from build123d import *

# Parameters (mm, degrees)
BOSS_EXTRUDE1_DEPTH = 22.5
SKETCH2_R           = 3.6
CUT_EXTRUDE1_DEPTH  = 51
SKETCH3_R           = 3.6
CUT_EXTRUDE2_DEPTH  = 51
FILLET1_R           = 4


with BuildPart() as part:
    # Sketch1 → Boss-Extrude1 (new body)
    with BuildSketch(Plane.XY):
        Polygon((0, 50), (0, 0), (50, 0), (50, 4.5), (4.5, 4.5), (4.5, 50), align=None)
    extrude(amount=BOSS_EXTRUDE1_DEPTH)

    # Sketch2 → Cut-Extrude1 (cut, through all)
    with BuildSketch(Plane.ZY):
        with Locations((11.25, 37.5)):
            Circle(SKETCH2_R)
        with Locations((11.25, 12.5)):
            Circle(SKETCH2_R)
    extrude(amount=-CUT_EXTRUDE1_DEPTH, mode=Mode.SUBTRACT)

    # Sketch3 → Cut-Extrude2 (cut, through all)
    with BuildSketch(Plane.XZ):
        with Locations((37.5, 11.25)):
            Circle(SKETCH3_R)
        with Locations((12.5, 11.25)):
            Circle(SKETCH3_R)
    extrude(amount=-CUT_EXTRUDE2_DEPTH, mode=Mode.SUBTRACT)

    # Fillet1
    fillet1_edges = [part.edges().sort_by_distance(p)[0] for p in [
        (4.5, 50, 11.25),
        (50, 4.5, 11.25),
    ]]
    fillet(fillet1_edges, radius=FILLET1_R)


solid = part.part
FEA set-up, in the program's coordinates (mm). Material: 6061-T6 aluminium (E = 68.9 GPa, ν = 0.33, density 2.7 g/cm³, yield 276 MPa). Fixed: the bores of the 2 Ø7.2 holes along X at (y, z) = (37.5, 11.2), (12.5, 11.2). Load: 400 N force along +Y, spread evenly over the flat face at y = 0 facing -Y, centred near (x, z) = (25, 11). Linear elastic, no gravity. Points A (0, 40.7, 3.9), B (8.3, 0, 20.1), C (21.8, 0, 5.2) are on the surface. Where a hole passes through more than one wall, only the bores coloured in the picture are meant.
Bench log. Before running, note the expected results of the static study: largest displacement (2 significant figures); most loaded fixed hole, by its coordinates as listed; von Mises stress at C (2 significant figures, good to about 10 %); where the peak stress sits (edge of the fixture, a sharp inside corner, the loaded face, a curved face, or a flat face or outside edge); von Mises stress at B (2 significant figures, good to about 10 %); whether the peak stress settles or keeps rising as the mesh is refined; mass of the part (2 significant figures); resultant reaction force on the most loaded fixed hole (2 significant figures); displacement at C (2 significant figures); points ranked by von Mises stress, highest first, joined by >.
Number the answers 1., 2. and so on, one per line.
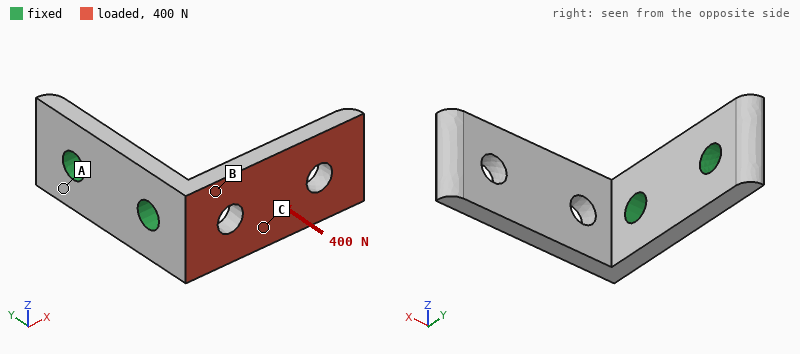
1. 0.76 mm
2. (12.5, 11.2)
3. 43 MPa
4. edge of the fixture
5. 110 MPa
6. keeps rising
7. 24 g
8. 380 N
9. 0.24 mm
10. B > C > A
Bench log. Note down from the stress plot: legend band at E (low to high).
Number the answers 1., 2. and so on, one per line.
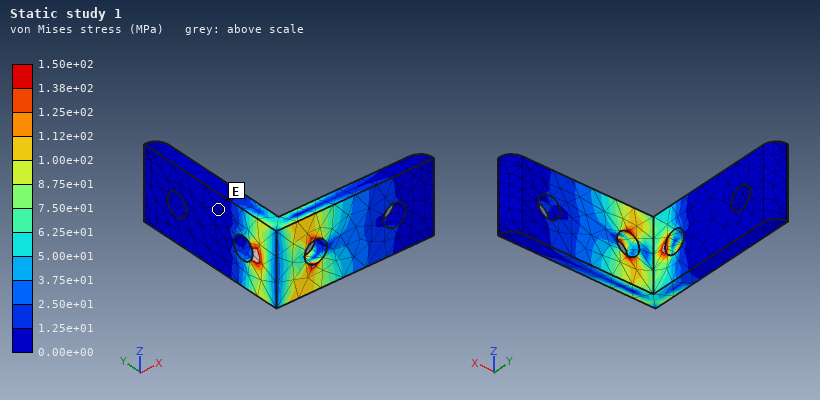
1. 0.00e+00 to 1.25e+01 MPa
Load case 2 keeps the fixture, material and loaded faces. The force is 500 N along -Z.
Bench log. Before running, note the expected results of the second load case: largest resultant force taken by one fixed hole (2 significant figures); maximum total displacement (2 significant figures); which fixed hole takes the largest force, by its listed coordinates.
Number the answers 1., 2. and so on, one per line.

1. 610 N
2. 0.20 mm
3. (12.5, 11.2)
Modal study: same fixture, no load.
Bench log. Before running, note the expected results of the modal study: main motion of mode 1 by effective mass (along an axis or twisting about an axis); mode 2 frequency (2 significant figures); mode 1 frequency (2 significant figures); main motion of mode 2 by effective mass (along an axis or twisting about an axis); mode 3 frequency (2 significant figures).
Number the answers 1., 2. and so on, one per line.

1. along Y
2. 2700 Hz
3. 1300 Hz
4. along Z
5. 6200 Hz
